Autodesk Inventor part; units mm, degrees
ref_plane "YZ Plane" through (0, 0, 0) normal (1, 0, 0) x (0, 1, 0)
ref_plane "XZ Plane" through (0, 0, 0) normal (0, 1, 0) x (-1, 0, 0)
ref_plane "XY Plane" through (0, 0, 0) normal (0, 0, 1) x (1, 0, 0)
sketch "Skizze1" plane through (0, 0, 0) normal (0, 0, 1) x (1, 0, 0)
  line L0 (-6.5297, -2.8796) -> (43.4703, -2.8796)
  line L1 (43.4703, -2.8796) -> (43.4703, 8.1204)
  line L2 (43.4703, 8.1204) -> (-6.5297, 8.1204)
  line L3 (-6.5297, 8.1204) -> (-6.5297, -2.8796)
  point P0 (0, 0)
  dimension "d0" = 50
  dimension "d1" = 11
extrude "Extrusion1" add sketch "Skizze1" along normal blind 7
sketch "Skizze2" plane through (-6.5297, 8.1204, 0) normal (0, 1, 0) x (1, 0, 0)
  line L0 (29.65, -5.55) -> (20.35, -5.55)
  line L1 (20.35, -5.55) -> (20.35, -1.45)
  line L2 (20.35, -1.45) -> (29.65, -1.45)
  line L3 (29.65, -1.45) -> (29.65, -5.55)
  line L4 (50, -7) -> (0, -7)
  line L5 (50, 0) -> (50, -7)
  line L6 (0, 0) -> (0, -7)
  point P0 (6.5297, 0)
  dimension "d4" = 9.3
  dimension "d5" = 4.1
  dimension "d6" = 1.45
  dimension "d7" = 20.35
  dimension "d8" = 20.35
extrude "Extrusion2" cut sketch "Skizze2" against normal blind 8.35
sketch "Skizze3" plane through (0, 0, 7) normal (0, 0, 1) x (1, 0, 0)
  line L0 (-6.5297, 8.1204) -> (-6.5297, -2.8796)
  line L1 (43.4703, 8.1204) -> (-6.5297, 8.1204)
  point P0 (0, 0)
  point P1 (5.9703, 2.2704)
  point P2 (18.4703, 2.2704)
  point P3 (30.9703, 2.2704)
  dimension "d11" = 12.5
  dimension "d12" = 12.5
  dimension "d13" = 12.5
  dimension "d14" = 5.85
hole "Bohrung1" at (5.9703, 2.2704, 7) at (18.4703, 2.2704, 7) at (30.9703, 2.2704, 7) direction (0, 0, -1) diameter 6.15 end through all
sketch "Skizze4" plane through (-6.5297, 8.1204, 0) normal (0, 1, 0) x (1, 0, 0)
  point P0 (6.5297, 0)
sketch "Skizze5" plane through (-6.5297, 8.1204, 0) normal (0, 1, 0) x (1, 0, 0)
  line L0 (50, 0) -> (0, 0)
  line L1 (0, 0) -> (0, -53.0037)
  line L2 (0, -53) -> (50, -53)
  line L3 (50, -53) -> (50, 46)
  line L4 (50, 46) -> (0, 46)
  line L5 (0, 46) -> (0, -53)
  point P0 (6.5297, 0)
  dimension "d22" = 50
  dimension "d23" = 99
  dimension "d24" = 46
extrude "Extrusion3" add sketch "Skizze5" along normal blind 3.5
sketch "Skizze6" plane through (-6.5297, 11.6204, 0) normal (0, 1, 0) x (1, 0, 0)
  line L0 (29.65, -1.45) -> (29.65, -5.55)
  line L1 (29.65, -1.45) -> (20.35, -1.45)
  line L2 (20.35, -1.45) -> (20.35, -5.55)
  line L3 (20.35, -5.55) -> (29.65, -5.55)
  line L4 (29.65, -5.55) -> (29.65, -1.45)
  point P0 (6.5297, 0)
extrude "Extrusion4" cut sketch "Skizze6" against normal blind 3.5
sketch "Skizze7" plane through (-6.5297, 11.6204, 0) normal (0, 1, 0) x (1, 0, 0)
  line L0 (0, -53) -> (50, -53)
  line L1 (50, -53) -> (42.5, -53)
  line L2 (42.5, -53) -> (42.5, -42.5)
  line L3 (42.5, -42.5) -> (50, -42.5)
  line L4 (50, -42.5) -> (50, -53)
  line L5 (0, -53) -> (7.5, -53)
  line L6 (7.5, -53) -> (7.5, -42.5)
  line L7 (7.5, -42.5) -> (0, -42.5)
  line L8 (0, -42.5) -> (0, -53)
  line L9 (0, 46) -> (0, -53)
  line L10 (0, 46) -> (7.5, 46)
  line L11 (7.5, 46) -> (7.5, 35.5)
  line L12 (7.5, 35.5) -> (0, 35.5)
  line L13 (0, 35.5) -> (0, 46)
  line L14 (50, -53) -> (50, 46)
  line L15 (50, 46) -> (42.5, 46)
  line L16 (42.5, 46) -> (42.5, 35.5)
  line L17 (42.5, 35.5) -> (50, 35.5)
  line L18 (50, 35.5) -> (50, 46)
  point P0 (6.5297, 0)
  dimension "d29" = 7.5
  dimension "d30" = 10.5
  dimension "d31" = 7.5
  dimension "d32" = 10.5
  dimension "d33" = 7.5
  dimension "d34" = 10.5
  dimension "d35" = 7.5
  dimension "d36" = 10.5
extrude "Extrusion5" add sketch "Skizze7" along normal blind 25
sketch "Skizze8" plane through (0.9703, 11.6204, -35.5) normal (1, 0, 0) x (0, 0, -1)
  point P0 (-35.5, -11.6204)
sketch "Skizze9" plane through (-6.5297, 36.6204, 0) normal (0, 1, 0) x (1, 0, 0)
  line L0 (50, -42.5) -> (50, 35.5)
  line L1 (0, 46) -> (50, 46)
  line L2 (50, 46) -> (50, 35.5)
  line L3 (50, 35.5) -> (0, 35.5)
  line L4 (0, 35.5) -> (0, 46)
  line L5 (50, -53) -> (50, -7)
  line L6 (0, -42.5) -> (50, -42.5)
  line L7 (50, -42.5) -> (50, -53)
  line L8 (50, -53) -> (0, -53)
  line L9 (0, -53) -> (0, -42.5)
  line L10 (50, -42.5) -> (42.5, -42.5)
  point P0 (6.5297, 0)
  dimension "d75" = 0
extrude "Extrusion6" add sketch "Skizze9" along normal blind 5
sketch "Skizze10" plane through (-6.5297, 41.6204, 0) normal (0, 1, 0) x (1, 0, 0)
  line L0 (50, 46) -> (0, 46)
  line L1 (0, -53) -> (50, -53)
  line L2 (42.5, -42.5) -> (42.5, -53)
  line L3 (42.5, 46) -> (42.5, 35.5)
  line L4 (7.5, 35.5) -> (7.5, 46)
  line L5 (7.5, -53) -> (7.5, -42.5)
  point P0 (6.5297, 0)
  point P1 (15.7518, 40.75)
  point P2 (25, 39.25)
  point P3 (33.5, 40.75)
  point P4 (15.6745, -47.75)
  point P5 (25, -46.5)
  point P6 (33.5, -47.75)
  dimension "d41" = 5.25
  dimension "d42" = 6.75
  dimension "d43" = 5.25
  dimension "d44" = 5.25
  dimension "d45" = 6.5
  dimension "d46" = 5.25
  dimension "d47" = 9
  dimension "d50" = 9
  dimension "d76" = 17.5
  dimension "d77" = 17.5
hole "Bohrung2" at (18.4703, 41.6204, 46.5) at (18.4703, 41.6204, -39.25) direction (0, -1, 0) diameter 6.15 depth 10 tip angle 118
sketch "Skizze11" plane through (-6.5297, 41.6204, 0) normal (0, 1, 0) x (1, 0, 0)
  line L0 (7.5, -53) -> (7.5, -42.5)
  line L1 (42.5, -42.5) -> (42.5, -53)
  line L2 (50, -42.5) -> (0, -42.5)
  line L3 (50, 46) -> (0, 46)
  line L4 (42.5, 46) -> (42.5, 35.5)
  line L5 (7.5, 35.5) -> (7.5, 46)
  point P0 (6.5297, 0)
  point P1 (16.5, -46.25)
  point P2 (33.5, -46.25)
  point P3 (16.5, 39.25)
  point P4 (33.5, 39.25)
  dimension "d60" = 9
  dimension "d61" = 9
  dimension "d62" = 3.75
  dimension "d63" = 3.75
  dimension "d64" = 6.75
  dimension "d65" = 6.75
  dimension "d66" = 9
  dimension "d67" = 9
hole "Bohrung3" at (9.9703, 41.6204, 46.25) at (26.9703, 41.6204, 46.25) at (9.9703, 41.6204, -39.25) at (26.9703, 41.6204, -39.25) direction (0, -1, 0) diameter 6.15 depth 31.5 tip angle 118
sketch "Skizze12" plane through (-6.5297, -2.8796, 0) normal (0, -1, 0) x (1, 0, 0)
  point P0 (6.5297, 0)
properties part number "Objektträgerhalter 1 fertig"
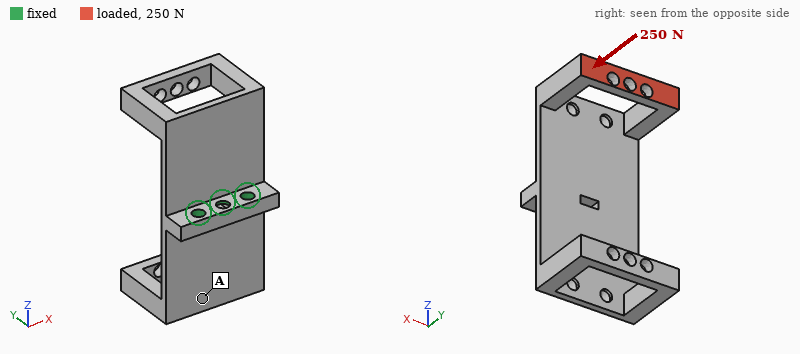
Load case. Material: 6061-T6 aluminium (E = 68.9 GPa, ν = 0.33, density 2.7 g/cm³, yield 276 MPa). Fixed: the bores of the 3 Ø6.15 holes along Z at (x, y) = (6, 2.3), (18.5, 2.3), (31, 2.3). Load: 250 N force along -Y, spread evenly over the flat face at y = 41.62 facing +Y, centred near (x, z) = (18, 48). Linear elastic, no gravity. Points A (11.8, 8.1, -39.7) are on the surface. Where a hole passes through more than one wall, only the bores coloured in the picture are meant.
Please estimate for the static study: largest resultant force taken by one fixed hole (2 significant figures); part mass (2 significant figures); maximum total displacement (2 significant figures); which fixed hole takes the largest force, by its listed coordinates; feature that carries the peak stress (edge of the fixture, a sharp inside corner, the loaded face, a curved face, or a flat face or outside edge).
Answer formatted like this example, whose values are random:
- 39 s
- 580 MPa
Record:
- 170 N
- 87 g
- 0.88 mm
- (18.5, 2.3)
- a flat face or outside edge
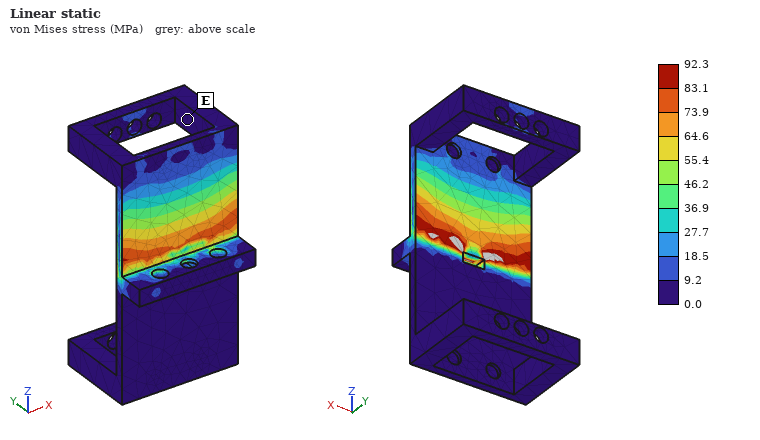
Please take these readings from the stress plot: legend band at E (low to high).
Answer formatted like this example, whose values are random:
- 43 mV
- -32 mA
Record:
- 0.0 to 9.2 MPa
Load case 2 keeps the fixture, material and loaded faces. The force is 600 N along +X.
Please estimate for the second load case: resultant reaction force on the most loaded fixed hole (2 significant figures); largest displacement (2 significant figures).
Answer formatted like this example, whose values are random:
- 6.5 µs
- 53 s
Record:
- 1.1 kN
- 1.0 mm
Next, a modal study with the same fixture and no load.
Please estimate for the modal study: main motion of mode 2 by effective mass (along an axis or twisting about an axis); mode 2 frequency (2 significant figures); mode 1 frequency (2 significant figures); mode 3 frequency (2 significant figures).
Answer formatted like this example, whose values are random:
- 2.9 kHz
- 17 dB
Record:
- along Y
- 600 Hz
- 570 Hz
- 1100 Hz
